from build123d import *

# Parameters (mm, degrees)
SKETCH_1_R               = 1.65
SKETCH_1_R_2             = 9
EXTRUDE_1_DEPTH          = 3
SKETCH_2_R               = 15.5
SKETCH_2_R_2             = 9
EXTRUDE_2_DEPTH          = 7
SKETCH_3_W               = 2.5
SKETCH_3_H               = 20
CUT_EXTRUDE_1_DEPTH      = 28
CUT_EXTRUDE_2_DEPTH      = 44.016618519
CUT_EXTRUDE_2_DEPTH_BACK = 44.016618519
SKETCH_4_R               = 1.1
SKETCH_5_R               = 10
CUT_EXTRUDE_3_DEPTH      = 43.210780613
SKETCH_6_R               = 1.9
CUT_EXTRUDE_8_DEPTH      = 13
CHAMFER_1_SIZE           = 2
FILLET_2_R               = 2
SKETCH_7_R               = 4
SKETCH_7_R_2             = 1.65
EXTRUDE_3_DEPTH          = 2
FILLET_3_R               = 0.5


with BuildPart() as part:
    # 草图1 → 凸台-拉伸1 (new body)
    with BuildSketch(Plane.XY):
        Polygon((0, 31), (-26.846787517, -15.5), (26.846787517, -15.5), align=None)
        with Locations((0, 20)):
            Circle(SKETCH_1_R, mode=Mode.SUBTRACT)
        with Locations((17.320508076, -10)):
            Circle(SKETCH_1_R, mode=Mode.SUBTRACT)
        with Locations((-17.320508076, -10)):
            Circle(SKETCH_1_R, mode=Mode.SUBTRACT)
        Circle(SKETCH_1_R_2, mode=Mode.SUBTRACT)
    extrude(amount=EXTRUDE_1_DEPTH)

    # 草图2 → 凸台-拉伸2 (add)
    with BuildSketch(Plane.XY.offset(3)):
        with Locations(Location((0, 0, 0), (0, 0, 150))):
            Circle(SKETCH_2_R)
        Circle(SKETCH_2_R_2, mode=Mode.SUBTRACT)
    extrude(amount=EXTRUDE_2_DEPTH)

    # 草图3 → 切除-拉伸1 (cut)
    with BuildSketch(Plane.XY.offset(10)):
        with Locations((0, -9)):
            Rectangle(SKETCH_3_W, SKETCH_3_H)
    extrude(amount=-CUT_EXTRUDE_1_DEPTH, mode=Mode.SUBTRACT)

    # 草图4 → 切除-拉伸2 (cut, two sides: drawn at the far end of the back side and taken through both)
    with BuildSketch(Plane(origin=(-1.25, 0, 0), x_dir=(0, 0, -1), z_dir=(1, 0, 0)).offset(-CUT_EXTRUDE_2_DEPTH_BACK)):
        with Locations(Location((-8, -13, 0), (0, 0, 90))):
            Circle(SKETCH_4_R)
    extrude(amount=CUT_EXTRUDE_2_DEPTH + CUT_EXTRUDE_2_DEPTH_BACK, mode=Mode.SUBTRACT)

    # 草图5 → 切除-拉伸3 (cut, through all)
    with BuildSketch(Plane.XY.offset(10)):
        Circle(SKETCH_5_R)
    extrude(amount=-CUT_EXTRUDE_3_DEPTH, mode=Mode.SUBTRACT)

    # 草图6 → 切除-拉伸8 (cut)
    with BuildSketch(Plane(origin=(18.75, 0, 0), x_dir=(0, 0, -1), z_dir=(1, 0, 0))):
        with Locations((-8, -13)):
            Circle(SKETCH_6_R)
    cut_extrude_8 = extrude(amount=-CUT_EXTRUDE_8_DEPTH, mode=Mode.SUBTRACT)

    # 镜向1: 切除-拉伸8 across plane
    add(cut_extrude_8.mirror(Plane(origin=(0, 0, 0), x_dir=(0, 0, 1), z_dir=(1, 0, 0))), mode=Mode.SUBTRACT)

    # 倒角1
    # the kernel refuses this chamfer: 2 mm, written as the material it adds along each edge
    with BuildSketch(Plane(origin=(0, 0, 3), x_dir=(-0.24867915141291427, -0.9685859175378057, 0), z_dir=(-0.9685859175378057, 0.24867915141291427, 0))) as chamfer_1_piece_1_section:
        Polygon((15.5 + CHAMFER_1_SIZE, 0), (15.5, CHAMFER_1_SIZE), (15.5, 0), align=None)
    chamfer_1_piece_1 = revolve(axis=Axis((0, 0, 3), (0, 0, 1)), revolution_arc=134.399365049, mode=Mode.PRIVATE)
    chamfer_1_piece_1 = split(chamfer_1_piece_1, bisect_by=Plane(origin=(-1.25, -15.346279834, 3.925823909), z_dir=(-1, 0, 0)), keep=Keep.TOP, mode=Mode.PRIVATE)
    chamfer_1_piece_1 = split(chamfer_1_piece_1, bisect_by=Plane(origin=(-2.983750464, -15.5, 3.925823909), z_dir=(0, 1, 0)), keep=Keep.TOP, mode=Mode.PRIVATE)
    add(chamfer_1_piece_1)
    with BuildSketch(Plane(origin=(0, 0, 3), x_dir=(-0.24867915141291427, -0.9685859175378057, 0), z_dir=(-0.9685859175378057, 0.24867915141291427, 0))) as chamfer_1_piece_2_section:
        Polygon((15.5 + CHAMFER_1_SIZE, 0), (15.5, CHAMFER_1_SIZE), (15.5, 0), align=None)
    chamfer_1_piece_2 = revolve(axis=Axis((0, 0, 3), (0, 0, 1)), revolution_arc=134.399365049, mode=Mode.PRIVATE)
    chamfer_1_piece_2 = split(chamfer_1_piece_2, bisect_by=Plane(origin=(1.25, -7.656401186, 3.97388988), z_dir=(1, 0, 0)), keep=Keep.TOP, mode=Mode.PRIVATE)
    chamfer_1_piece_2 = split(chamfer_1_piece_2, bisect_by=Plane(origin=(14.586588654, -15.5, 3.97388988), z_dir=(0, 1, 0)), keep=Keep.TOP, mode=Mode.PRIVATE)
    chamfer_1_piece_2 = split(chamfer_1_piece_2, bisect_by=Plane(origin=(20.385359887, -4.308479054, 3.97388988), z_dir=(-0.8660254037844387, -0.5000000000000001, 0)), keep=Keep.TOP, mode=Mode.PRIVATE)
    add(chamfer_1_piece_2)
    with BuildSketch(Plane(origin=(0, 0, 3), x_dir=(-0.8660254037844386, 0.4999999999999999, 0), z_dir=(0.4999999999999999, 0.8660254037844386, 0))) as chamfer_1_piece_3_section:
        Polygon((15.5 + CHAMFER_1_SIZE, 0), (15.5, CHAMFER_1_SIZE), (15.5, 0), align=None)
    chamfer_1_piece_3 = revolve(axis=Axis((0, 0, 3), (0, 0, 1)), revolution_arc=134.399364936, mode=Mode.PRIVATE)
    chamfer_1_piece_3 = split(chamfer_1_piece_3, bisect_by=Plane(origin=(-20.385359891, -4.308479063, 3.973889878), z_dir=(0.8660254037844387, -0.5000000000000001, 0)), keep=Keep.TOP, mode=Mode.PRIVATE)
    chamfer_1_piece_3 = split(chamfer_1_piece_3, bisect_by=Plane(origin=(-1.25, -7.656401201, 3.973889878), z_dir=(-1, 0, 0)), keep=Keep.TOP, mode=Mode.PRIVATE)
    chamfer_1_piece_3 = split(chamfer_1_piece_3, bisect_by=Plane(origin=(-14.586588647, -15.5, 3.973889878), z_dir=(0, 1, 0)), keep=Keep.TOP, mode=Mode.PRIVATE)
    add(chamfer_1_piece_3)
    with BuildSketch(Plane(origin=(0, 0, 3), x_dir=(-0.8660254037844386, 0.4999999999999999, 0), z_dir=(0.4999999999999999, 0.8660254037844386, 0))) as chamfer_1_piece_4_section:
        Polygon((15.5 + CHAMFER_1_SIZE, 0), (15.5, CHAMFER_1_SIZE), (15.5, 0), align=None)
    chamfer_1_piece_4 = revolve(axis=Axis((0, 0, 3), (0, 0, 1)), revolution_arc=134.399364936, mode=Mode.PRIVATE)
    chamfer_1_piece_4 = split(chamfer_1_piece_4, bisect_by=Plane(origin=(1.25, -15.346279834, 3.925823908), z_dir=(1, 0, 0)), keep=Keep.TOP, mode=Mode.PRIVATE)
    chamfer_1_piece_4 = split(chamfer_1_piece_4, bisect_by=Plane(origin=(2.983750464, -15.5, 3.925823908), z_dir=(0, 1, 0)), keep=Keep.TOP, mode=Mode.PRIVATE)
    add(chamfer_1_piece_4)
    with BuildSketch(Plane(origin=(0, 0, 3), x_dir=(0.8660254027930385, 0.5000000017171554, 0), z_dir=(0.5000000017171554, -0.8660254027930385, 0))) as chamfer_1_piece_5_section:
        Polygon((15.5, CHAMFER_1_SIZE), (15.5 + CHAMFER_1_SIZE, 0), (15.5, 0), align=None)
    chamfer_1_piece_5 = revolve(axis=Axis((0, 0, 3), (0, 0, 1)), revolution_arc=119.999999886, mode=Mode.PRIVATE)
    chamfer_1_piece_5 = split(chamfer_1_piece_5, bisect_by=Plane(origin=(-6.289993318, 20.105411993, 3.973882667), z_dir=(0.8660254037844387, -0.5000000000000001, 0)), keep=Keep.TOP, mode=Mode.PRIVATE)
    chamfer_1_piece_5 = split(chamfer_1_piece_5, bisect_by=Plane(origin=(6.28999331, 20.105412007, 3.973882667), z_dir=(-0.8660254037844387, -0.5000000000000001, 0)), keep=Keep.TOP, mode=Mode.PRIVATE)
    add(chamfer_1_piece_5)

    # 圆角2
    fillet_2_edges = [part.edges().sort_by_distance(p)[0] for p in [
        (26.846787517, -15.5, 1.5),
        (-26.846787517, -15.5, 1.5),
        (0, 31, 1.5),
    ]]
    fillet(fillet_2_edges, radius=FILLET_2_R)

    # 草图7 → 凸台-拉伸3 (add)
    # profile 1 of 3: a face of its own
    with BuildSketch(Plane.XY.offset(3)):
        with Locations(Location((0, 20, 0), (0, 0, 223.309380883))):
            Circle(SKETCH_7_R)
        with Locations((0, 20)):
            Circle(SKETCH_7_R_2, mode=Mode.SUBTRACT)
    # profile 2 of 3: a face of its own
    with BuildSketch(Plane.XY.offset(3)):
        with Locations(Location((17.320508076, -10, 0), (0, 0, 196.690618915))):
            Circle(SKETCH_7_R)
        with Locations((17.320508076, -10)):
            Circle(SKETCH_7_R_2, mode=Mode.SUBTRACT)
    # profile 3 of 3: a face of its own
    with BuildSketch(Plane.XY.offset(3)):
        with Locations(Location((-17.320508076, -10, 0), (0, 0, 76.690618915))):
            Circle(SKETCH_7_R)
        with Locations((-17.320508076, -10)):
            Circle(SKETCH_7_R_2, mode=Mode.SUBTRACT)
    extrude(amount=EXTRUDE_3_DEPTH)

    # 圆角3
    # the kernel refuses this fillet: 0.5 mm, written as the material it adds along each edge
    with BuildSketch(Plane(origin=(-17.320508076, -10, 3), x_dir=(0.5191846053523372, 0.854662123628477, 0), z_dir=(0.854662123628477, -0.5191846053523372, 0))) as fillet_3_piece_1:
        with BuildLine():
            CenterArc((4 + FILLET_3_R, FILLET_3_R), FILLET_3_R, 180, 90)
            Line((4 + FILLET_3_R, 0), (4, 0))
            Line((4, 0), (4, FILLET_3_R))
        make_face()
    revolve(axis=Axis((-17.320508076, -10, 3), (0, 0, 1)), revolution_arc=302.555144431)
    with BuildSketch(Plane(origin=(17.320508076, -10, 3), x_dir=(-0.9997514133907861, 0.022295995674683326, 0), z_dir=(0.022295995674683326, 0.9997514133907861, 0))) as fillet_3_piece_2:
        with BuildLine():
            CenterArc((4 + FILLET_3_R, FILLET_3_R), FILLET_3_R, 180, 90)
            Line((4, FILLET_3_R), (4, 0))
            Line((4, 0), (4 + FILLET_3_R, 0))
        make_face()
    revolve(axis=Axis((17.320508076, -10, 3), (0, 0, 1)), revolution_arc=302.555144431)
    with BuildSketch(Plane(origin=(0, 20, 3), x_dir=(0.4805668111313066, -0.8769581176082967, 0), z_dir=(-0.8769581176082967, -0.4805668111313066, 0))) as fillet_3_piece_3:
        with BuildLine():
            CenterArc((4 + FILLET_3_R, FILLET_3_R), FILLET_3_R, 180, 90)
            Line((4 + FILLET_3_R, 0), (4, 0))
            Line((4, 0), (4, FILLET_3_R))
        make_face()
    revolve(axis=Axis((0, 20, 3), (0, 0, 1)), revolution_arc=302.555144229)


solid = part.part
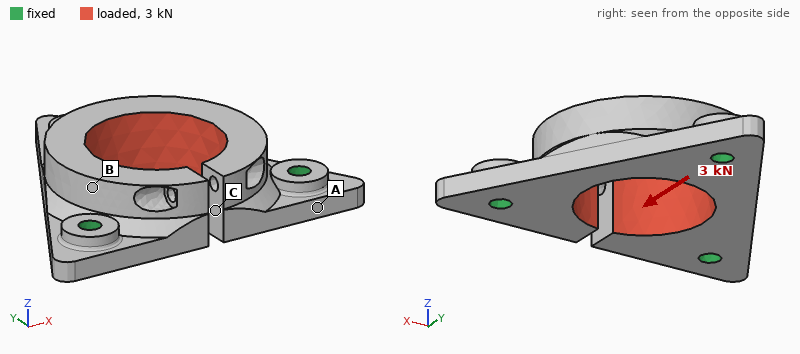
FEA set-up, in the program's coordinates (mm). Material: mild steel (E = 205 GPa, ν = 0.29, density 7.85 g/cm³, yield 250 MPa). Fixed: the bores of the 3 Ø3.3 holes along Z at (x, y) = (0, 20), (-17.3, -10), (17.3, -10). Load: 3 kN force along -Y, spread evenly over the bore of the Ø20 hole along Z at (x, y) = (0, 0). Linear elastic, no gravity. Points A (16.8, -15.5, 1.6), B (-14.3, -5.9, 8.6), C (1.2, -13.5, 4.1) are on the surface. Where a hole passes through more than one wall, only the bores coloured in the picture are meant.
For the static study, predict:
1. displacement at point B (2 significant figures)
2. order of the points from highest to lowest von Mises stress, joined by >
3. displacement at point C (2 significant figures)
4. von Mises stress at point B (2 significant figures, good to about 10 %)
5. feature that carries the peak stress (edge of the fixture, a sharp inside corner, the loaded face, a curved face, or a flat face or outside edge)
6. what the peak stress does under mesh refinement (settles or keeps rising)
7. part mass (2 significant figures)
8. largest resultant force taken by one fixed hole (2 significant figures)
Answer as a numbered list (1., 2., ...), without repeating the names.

1. 2.2 µm
2. A > B > C
3. 7.9 µm
4. 15 MPa
5. edge of the fixture
6. keeps rising
7. 47 g
8. 1.1 kN
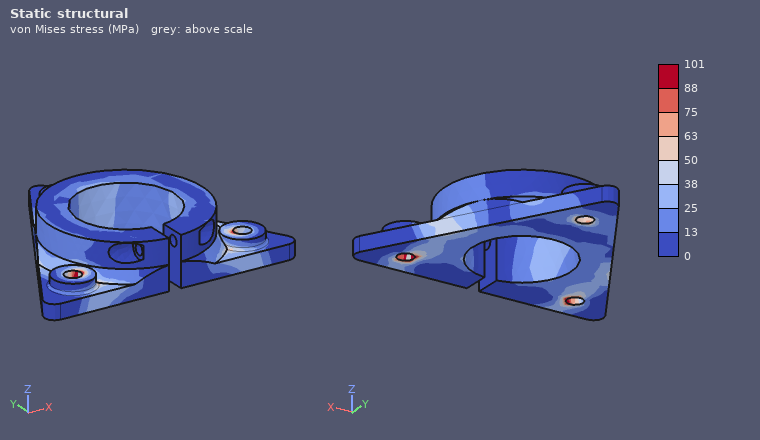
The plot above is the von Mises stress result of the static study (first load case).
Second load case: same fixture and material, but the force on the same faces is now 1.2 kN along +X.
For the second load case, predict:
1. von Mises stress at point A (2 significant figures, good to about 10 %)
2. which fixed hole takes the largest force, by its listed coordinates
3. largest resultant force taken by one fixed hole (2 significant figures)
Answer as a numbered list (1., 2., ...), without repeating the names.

1. 7.1 MPa
2. (0, 20)
3. 530 N
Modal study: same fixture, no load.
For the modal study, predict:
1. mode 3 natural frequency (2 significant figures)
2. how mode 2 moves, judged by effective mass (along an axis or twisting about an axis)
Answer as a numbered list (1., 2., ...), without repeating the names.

1. 16 kHz
2. along Z
